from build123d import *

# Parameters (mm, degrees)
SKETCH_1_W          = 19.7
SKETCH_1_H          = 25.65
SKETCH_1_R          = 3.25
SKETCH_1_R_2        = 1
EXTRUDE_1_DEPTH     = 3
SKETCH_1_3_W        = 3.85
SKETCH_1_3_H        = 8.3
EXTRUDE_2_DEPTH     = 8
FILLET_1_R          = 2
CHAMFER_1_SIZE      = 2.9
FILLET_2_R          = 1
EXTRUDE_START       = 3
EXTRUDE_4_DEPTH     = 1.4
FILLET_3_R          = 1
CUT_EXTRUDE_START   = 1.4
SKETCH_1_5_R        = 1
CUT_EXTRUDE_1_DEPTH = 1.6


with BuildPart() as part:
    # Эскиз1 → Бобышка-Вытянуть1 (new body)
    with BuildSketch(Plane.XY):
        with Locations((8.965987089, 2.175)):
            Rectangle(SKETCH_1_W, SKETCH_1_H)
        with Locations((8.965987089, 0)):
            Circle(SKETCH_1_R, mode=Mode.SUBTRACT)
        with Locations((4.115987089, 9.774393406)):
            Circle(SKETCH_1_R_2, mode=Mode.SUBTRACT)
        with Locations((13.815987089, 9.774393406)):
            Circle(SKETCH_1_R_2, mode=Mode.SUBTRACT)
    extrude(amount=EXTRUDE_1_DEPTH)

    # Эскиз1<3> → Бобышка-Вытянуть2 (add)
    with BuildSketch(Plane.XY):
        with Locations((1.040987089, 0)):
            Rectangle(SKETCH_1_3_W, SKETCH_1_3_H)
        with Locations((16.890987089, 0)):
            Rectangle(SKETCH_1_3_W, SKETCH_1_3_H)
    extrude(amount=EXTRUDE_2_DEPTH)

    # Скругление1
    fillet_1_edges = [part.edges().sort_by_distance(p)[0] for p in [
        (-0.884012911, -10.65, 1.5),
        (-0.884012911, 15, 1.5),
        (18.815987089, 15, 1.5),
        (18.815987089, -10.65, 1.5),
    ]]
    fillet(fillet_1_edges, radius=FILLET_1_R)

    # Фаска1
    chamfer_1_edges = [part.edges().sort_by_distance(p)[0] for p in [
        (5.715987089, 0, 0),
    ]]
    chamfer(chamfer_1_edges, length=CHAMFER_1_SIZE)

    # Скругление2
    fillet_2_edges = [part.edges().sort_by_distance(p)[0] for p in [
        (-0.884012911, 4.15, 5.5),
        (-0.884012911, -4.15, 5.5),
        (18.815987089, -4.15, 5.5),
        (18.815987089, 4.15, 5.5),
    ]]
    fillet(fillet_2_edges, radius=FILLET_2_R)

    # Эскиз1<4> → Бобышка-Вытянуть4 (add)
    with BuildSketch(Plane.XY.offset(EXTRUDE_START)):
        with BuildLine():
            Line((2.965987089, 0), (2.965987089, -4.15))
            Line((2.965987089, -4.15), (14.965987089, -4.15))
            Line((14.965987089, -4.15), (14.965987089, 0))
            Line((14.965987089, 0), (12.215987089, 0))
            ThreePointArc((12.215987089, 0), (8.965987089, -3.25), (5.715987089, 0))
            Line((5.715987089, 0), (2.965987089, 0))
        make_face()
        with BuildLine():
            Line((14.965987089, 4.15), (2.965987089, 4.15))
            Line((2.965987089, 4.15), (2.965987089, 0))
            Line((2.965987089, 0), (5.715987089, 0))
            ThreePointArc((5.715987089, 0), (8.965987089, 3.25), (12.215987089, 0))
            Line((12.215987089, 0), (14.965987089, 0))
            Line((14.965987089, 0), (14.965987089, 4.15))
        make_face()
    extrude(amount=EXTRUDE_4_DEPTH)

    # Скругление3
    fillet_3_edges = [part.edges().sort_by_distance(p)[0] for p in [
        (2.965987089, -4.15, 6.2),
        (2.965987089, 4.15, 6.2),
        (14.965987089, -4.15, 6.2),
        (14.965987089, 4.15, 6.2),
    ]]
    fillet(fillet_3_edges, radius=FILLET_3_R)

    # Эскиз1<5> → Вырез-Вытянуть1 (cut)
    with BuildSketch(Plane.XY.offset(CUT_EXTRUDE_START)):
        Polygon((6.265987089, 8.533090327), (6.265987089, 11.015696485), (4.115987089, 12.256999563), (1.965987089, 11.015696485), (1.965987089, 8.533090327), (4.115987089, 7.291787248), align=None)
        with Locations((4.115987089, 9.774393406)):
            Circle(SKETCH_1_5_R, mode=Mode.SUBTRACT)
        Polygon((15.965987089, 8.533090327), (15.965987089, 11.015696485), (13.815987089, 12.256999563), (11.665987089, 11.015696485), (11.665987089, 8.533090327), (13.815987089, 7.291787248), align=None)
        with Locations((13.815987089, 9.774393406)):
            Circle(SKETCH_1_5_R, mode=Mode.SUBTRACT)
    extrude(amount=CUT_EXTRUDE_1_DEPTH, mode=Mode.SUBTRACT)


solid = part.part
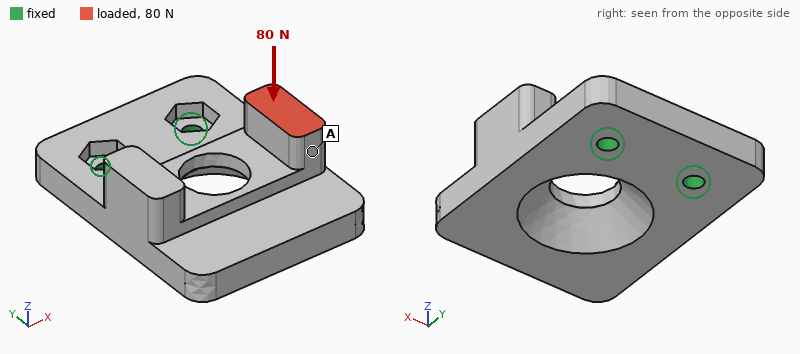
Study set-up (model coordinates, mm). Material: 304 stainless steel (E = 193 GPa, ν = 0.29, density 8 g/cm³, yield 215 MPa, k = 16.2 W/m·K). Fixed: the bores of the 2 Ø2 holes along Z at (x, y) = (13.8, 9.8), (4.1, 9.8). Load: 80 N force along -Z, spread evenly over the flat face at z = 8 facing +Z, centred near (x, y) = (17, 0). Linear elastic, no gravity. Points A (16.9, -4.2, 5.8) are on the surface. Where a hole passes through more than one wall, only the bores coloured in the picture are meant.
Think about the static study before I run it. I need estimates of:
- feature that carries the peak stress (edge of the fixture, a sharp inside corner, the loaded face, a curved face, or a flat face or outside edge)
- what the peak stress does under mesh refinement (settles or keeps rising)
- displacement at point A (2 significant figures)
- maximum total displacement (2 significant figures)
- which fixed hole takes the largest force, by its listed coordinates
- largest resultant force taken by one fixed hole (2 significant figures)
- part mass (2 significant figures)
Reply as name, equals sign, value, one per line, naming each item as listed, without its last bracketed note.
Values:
feature that carries the peak stress = edge of the fixture
what the peak stress does under mesh refinement = keeps rising
displacement at point A = 18 µm
maximum total displacement = 25 µm
which fixed hole takes the largest force, by its listed coordinates = (13.8, 9.8)
largest resultant force taken by one fixed hole = 95 N
part mass = 13 g
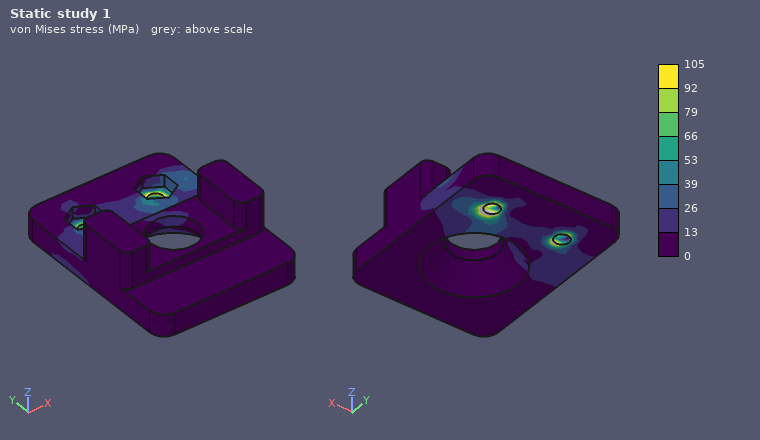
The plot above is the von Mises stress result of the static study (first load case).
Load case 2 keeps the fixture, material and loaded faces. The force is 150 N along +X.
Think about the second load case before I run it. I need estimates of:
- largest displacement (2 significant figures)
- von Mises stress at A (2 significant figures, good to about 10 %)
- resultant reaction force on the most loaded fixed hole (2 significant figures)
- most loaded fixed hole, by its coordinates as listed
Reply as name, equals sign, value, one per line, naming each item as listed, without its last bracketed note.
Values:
largest displacement = 10 µm
von Mises stress at A = 12 MPa
resultant reaction force on the most loaded fixed hole = 200 N
most loaded fixed hole, by its coordinates as listed = (4.1, 9.8)
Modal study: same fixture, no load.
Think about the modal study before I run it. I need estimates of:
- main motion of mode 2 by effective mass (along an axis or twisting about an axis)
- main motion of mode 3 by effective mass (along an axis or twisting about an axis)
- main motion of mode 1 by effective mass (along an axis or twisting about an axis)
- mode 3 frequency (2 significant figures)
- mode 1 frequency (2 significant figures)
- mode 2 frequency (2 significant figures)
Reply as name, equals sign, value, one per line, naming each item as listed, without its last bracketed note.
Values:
main motion of mode 2 by effective mass = twisting about Y
main motion of mode 3 by effective mass = along X
main motion of mode 1 by effective mass = along Z
mode 3 frequency = 14 kHz
mode 1 frequency = 3500 Hz
mode 2 frequency = 8900 Hz
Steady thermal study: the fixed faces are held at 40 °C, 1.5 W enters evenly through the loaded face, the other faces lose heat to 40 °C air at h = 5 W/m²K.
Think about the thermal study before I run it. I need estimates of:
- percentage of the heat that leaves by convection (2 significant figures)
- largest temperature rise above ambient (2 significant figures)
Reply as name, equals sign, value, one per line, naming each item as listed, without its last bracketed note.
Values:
percentage of the heat that leaves by convection = 7.1 %
largest temperature rise above ambient = 42 K
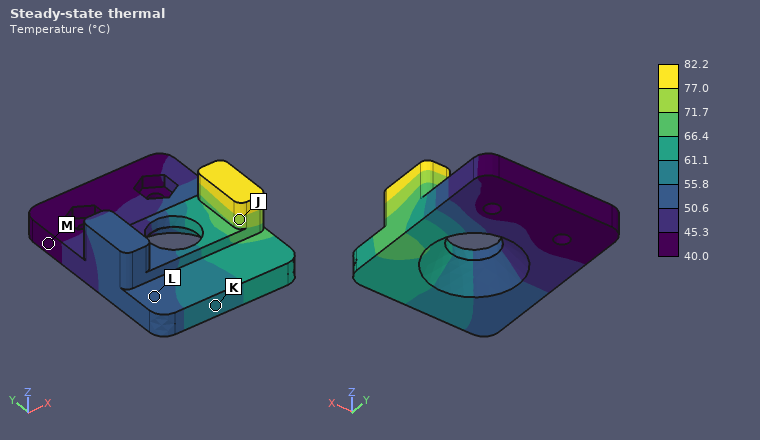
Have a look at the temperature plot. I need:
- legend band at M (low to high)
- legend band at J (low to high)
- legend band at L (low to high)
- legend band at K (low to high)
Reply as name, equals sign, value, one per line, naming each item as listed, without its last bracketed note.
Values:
legend band at M = 40.0 to 45.3 °C
legend band at J = 71.7 to 77.0 °C
legend band at L = 50.6 to 55.8 °C
legend band at K = 55.8 to 61.1 °C
